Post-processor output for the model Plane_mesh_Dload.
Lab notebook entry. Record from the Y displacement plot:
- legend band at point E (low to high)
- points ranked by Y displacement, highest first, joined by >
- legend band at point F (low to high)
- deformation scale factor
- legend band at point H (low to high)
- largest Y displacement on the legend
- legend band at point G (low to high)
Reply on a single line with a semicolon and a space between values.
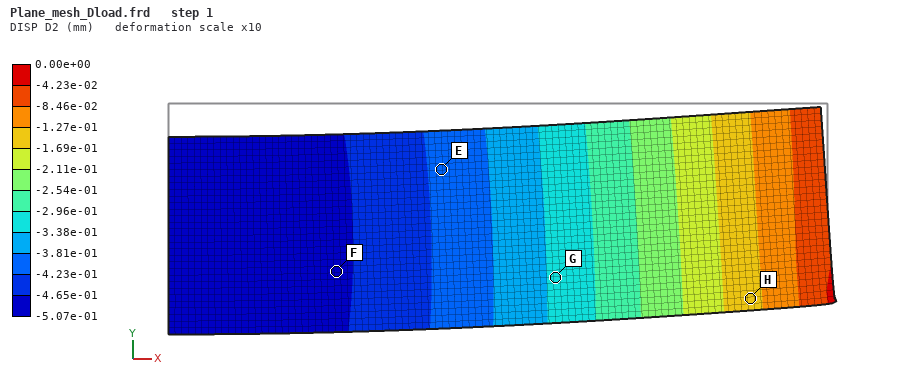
-4.23e-01 to -3.81e-01 mm; H > G > E > F; -5.07e-01 to -4.65e-01 mm; 10; -1.69e-01 to -1.27e-01 mm; 0.00e+00 mm; -3.38e-01 to -2.96e-01 mm
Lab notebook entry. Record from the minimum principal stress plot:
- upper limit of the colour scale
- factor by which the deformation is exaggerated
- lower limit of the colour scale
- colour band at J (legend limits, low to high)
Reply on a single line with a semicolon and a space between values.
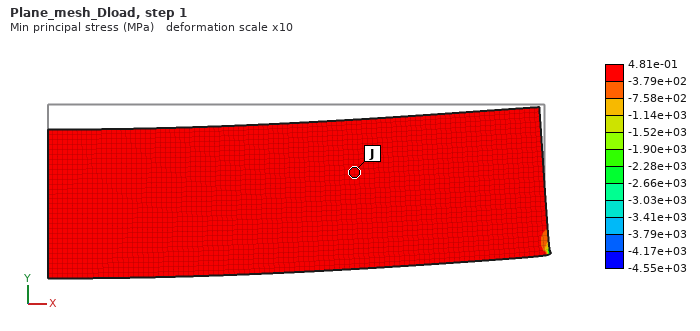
4.81e-01 MPa; 10; -4.55e+03 MPa; -3.79e+02 to 4.81e-01 MPa
